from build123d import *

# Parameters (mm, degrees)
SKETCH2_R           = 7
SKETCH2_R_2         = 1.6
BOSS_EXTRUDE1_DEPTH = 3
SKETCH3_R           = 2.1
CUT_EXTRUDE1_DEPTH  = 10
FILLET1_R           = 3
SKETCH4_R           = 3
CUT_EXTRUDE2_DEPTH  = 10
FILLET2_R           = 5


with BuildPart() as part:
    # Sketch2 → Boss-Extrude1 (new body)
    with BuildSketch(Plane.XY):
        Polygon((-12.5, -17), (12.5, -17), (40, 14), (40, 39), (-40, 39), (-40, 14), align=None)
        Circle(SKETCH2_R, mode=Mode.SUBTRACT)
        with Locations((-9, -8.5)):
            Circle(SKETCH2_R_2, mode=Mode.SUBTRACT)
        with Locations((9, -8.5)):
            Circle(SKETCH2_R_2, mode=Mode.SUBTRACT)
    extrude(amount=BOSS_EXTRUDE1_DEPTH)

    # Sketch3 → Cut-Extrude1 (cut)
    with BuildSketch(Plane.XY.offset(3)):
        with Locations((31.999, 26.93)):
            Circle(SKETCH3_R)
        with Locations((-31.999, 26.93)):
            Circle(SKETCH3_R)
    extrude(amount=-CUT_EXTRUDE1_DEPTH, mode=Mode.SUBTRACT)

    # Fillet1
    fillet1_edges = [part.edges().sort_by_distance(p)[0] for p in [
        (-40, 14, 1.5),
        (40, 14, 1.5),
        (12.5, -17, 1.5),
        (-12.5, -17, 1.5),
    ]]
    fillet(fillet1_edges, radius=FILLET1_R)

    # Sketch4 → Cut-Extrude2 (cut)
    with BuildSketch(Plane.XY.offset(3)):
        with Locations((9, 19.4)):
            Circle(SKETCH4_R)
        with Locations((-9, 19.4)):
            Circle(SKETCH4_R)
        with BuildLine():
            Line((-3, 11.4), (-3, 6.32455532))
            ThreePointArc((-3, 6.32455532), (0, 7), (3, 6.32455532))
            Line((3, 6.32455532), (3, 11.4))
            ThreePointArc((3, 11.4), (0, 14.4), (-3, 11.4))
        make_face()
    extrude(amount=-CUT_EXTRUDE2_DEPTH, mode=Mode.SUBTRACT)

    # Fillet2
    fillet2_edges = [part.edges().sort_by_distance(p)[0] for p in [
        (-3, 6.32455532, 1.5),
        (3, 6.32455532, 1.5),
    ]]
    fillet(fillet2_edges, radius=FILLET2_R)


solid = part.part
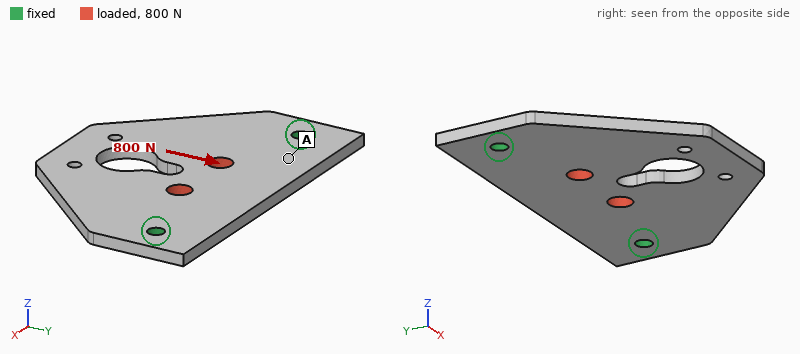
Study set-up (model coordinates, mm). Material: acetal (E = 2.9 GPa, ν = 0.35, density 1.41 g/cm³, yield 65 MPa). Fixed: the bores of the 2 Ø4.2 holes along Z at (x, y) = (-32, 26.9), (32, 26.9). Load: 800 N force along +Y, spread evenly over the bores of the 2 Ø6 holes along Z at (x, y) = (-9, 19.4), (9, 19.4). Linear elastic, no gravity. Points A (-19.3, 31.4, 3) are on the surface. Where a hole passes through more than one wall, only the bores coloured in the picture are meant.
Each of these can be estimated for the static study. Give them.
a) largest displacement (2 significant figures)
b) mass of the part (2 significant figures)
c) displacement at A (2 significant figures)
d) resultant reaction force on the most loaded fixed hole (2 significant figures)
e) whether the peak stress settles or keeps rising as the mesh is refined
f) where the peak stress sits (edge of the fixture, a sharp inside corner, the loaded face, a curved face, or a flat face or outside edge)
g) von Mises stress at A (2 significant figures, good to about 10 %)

0.18 mm
14 g
0.096 mm
410 N
keeps rising
edge of the fixture
5.3 MPa
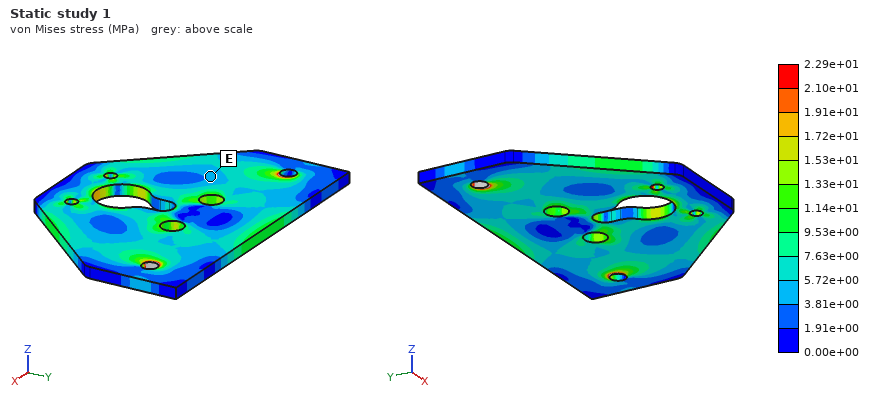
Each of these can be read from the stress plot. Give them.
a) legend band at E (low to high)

3.81e+00 to 5.72e+00 MPa
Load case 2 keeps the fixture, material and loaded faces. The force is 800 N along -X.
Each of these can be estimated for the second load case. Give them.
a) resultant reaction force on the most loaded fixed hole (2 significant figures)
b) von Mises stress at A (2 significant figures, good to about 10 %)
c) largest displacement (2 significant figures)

410 N
4.7 MPa
90 µm
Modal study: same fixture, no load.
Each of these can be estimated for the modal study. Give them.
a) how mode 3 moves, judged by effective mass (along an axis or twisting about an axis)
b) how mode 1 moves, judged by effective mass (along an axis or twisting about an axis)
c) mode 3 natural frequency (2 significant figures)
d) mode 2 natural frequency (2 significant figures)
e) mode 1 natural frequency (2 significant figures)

along Z
along Z
1100 Hz
1000 Hz
380 Hz
